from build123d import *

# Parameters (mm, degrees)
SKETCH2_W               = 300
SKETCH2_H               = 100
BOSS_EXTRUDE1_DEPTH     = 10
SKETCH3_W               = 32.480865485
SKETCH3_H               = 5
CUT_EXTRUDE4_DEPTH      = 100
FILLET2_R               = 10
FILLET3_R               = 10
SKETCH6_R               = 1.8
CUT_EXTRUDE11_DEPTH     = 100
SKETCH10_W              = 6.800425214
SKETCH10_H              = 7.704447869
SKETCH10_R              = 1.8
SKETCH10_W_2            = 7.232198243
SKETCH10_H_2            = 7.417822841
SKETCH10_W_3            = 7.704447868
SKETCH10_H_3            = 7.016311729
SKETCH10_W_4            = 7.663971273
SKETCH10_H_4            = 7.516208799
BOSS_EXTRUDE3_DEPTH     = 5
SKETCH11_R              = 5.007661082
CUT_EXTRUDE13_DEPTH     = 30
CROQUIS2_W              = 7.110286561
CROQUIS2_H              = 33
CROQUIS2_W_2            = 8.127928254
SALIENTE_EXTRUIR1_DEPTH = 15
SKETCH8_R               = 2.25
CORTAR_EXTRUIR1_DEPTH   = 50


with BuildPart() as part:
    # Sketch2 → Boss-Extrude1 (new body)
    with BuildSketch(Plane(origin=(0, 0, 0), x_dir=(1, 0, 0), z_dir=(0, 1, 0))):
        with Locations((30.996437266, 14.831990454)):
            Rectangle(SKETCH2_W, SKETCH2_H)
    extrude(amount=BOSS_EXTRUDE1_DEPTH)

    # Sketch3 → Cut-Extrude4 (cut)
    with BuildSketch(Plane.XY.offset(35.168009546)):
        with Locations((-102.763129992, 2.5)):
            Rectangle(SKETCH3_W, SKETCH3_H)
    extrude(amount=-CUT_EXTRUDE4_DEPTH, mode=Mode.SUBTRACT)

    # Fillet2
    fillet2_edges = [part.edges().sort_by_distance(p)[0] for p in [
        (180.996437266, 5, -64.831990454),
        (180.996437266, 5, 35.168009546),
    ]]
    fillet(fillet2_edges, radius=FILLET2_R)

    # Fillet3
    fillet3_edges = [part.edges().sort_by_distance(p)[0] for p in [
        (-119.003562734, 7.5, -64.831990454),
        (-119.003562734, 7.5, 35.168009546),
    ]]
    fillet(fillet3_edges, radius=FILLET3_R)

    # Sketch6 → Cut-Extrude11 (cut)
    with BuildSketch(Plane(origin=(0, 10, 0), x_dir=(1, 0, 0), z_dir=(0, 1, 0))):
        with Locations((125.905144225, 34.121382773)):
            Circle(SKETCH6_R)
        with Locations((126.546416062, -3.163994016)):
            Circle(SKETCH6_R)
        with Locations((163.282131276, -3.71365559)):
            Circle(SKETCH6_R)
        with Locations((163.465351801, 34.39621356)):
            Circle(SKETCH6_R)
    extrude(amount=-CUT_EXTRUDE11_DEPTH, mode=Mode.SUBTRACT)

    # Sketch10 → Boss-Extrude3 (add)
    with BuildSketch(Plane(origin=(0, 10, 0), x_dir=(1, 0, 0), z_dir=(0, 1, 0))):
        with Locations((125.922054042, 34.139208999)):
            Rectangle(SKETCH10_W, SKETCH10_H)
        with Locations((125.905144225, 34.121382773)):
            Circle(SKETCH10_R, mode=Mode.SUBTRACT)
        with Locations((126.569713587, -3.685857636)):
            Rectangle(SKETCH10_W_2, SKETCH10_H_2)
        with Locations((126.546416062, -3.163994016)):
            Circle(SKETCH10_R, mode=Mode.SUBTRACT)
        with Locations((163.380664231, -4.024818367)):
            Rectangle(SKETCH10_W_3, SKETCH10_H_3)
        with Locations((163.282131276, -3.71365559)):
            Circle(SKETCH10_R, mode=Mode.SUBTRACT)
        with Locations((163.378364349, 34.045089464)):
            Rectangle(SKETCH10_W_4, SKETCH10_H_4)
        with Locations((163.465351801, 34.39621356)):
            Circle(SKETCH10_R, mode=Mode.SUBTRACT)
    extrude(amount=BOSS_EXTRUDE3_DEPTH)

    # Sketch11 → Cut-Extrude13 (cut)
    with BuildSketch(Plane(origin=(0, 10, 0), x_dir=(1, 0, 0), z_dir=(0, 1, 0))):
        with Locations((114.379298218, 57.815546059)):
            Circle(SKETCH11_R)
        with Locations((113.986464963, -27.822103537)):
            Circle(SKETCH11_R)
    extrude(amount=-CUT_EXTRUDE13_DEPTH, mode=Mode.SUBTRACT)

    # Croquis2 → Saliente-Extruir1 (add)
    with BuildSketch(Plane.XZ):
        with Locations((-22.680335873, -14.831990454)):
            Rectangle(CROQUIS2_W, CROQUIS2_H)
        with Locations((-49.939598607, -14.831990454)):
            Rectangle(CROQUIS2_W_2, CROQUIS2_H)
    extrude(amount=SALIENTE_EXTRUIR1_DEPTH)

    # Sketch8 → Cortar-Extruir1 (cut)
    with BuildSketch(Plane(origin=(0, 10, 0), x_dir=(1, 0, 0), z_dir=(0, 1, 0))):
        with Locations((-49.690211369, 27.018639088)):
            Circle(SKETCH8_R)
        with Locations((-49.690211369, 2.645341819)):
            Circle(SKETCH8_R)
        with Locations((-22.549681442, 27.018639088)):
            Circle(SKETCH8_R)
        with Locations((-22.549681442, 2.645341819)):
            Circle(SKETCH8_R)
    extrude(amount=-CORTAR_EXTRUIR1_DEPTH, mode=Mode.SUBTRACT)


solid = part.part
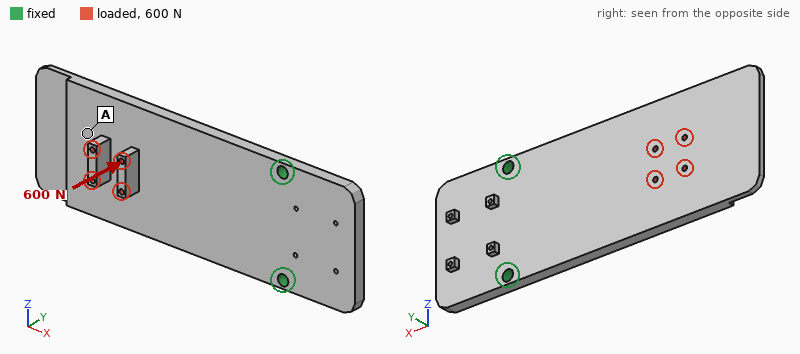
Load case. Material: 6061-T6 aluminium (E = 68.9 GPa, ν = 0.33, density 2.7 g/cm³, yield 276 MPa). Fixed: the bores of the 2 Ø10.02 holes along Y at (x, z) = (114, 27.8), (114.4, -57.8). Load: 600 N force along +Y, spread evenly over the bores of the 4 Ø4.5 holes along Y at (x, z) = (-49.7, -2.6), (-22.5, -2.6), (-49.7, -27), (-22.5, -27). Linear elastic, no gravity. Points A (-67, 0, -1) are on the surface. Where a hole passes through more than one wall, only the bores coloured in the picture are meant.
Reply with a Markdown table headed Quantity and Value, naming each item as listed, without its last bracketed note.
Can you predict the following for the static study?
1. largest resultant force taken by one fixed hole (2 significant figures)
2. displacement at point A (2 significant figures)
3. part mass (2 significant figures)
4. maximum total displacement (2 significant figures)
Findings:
| Quantity | Value |
|---|---|
| largest resultant force taken by one fixed hole | 310 N |
| displacement at point A | 1.7 mm |
| part mass | 780 g |
| maximum total displacement | 2.3 mm |
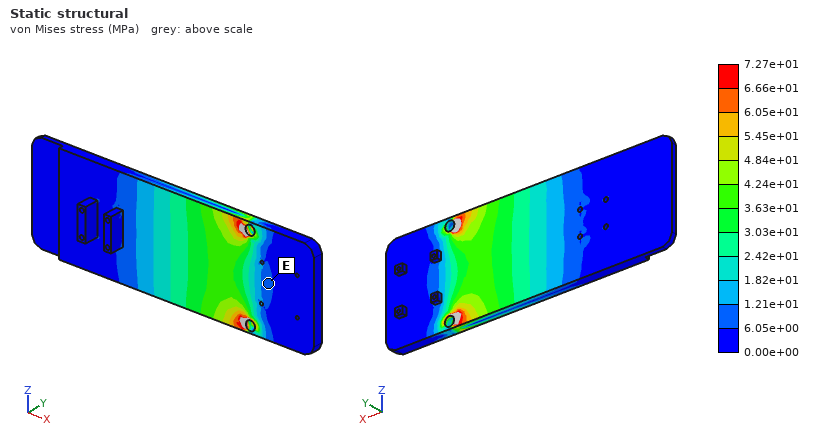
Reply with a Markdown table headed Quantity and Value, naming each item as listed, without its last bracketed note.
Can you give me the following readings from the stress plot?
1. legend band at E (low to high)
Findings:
| Quantity | Value |
|---|---|
| legend band at E | 6.05e+00 to 1.21e+01 MPa |
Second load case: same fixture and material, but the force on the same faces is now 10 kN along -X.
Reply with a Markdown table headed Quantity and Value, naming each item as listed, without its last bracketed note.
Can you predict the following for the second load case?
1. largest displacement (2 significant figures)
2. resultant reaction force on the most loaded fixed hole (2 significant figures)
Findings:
| Quantity | Value |
|---|---|
| largest displacement | 3.2 mm |
| resultant reaction force on the most loaded fixed hole | 5.1 kN |
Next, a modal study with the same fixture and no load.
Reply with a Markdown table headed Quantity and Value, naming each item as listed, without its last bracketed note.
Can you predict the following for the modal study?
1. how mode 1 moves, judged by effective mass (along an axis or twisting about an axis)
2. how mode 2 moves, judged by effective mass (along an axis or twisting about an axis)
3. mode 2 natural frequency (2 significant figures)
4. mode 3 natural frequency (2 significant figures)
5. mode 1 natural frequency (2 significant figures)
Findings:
| Quantity | Value |
|---|---|
| how mode 1 moves, judged by effective mass | along Y |
| how mode 2 moves, judged by effective mass | twisting about X |
| mode 2 natural frequency | 780 Hz |
| mode 3 natural frequency | 980 Hz |
| mode 1 natural frequency | 160 Hz |
